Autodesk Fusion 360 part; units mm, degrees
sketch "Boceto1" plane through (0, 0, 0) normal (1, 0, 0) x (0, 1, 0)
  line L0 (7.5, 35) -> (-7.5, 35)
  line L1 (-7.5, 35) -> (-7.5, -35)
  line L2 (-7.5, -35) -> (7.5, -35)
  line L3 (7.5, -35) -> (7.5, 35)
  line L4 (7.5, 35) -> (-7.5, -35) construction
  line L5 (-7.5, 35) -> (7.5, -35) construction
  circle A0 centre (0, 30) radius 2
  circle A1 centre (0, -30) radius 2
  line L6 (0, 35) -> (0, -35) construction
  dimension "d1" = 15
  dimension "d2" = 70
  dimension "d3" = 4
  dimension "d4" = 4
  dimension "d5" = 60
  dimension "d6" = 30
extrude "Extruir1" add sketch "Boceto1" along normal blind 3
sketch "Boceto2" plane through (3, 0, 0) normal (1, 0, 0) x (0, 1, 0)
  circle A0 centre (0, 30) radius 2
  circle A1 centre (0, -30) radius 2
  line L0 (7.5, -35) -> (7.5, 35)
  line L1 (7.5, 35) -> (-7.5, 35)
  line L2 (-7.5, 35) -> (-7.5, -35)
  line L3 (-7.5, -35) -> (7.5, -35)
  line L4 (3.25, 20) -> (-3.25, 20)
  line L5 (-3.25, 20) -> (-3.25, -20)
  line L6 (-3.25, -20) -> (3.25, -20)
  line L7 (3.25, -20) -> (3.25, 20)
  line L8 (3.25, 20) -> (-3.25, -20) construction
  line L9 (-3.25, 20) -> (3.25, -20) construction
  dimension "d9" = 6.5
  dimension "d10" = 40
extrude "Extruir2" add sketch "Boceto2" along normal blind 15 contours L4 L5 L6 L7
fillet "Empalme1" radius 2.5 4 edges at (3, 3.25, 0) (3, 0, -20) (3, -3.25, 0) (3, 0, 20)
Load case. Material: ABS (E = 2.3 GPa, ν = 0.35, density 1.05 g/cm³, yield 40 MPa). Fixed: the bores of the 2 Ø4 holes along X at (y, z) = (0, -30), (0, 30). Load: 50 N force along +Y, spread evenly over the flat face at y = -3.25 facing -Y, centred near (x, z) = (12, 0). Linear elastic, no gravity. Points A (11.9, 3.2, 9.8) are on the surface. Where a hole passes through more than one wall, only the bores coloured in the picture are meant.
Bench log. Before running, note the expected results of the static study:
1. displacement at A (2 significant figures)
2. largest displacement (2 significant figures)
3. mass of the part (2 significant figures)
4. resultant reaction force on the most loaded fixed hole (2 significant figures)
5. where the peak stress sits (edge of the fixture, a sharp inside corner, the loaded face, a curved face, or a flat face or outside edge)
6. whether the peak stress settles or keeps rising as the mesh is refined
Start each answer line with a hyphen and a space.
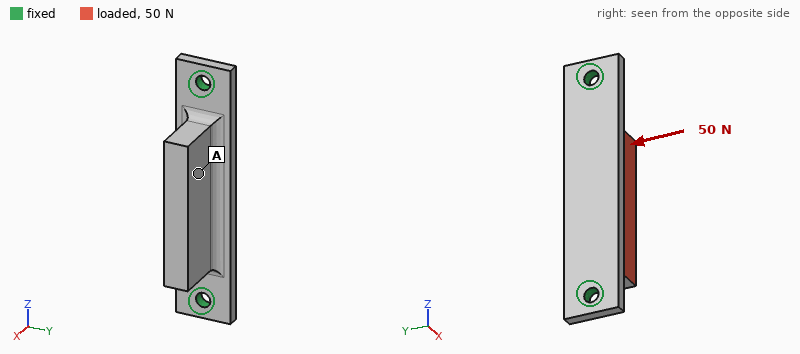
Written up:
- 0.26 mm
- 0.39 mm
- 7.5 g
- 25 N
- edge of the fixture
- keeps rising
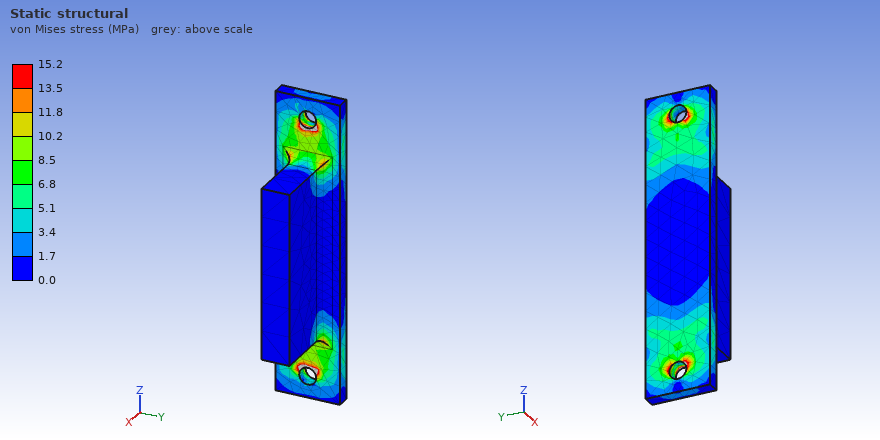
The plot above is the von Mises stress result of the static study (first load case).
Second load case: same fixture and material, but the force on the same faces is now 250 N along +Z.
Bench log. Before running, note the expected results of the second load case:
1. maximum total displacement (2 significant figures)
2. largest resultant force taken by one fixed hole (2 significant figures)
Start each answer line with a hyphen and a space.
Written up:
- 0.12 mm
- 140 N
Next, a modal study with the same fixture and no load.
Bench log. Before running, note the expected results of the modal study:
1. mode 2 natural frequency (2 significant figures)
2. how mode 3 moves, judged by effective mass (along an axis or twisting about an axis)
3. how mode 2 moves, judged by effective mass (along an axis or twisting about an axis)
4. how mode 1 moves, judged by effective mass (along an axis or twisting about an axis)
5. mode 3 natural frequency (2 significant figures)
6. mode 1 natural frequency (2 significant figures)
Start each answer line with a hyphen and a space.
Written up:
- 2100 Hz
- along Y
- along X
- along Y
- 3200 Hz
- 1100 Hz
